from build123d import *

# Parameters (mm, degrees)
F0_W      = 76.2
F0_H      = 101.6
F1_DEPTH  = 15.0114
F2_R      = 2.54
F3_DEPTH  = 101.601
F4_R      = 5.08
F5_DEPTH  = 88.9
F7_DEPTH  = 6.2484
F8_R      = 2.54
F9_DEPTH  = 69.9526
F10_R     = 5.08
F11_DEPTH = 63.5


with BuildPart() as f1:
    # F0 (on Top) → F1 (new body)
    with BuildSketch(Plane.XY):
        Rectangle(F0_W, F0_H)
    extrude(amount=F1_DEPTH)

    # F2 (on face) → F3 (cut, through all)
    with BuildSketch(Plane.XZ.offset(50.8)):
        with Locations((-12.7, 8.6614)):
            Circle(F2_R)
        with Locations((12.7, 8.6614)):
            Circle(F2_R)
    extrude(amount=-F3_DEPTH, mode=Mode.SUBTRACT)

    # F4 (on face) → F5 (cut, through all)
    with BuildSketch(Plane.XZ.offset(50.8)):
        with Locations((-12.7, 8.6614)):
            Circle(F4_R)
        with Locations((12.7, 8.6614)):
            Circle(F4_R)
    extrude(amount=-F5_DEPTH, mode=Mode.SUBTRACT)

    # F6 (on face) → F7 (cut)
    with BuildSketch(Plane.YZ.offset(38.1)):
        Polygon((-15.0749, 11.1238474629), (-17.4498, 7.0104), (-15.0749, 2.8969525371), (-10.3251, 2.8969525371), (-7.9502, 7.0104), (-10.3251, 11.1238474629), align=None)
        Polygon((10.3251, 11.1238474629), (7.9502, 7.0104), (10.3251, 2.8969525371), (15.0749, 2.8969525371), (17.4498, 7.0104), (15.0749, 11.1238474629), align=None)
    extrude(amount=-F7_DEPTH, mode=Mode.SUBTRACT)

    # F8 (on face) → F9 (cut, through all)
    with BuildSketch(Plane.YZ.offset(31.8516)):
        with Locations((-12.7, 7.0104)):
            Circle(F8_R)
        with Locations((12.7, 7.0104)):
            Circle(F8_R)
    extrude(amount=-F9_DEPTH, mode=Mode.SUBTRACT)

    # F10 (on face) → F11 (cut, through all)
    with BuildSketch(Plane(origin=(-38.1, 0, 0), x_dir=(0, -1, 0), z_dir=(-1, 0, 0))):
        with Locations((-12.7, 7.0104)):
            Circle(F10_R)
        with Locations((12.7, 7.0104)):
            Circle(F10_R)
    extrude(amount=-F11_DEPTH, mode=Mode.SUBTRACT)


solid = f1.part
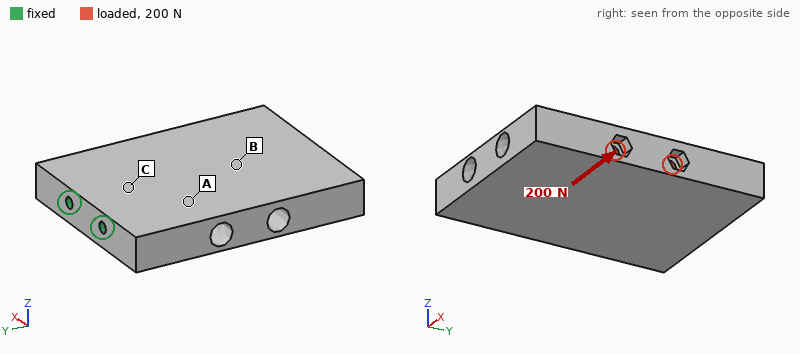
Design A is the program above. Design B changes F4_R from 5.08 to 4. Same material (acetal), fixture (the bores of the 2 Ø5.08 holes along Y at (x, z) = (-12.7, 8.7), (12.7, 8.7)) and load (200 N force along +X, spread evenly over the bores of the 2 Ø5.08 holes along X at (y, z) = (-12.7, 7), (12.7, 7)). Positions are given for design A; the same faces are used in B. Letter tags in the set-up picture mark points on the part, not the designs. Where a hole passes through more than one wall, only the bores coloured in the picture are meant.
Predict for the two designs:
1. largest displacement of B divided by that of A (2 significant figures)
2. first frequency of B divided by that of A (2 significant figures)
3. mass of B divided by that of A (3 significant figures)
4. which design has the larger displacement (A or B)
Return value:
0.89
1.00
1.05
A
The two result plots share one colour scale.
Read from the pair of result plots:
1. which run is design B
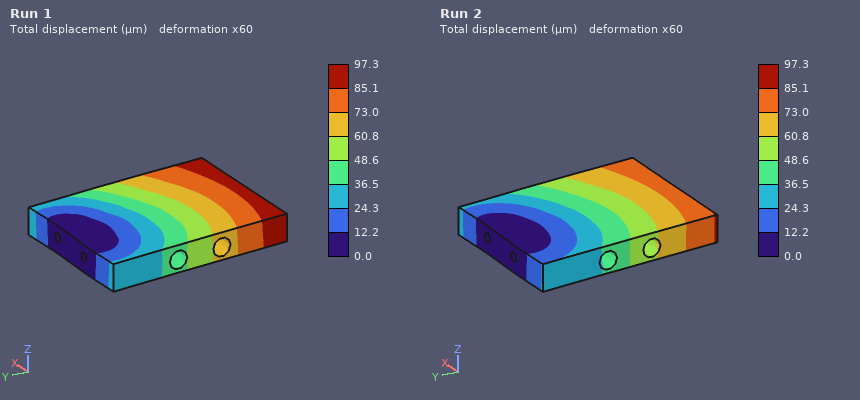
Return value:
Run 2
